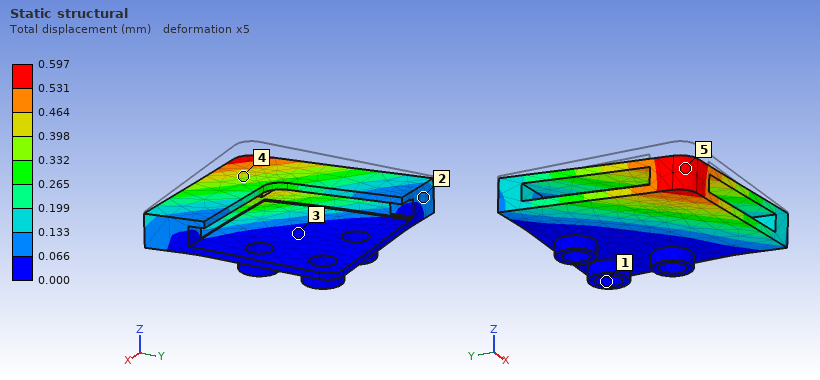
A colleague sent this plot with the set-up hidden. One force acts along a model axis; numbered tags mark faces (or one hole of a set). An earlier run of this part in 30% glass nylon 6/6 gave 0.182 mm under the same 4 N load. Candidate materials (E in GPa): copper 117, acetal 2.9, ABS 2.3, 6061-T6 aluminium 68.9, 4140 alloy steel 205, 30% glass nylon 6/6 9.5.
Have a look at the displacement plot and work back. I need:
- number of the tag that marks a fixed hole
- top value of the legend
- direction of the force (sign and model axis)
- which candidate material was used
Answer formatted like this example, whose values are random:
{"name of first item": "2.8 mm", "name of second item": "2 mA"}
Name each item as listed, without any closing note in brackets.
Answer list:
{"number of the tag that marks a fixed hole": "1", "top value of the legend": "0.597 mm", "direction of the force": "-Z", "which candidate material was used": "acetal"}
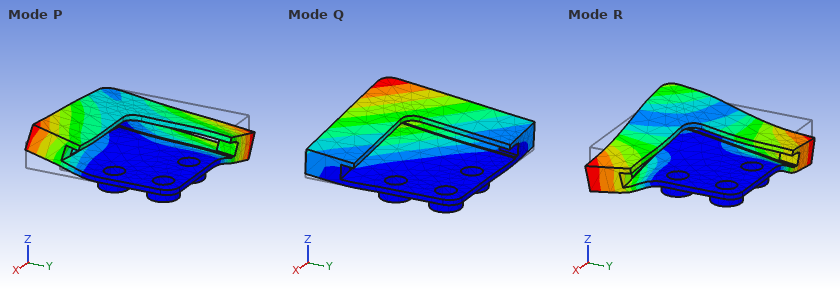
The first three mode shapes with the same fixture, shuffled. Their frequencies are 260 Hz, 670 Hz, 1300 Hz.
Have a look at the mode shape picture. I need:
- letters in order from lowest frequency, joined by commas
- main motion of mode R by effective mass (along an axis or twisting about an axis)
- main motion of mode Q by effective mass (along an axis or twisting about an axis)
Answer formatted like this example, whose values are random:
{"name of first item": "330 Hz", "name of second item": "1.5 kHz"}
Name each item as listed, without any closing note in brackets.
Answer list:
{"letters in order from lowest frequency, joined by commas": "Q, P, R", "main motion of mode R by effective mass": "along Z", "main motion of mode Q by effective mass": "along Z"}
